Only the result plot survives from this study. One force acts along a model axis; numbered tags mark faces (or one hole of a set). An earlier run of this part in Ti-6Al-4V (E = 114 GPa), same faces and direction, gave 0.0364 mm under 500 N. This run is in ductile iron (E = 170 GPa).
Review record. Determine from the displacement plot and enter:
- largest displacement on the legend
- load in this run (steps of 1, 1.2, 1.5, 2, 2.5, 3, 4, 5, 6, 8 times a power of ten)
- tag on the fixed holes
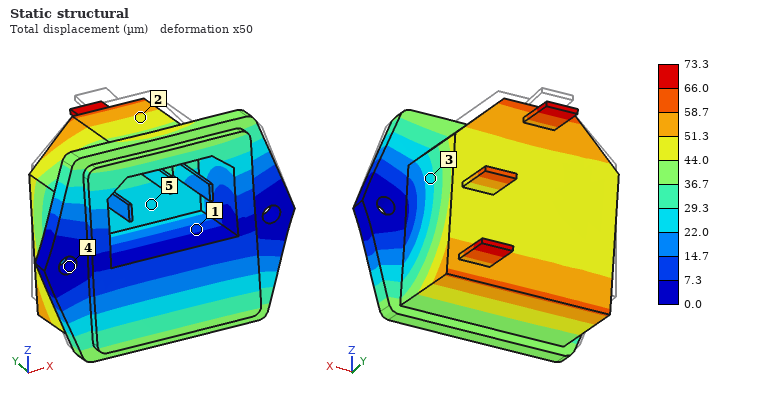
73.3 µm
1.5 kN
4
